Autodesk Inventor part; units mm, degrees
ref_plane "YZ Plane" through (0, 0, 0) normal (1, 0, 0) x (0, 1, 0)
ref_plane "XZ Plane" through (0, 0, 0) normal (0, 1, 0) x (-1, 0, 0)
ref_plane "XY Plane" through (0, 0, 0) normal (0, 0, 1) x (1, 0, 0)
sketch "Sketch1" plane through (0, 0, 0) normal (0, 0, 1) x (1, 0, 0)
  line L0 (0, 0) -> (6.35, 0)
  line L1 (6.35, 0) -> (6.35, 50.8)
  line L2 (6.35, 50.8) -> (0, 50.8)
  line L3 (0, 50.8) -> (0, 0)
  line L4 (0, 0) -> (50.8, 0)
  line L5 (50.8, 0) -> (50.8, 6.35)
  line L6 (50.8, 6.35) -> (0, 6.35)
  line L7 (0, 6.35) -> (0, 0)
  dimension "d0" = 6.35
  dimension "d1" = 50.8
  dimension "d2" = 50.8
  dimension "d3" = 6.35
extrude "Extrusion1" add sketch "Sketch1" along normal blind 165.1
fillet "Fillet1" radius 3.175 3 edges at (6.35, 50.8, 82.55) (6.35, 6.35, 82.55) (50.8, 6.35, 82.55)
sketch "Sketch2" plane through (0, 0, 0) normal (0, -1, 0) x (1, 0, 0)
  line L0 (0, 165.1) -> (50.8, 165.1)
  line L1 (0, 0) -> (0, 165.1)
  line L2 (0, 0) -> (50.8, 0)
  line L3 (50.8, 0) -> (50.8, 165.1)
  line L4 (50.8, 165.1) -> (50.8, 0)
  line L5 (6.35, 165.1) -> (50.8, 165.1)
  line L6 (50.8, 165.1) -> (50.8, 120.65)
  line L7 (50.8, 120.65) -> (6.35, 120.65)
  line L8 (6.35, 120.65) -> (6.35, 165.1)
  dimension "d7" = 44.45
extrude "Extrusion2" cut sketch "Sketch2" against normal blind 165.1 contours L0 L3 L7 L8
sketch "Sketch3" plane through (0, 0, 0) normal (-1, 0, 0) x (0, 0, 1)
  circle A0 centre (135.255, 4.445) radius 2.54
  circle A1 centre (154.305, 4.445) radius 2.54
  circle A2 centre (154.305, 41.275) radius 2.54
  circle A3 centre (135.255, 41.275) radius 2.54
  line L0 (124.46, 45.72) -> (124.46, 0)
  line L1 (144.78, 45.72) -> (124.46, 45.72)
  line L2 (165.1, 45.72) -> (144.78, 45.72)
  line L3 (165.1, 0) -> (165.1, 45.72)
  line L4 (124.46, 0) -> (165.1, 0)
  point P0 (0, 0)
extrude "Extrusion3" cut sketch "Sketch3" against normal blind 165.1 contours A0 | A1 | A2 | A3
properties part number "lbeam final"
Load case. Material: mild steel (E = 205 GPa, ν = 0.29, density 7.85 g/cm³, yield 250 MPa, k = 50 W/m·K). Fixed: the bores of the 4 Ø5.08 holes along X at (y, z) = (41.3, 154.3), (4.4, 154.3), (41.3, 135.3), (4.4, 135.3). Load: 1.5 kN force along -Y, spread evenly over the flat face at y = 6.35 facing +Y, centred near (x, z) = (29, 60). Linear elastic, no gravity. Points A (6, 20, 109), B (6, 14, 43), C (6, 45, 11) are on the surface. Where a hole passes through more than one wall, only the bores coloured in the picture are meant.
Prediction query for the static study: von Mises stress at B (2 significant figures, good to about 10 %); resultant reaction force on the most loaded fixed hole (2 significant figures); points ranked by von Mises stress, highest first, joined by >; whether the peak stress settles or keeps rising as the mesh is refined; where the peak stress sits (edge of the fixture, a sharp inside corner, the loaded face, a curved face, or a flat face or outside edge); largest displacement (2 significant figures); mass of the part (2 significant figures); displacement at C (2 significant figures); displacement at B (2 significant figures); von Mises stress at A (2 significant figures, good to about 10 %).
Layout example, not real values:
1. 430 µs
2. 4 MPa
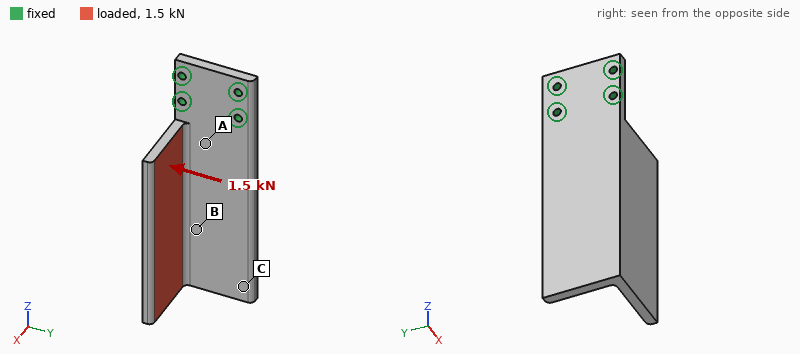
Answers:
1. 32 MPa
2. 2.9 kN
3. A > B > C
4. keeps rising
5. edge of the fixture
6. 0.38 mm
7. 680 g
8. 0.064 mm
9. 0.083 mm
10. 76 MPa
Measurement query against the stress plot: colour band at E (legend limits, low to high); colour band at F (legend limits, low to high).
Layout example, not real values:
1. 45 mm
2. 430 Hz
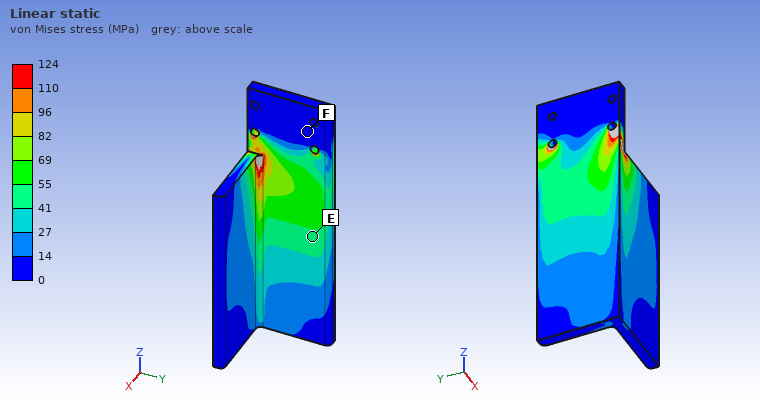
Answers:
1. 41 to 55 MPa
2. 0 to 14 MPa
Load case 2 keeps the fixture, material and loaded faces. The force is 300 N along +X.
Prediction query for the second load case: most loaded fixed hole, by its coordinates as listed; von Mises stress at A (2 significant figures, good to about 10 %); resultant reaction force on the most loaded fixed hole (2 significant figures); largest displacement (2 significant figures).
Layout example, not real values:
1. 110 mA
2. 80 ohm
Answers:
1. (4.4, 135.3)
2. 30 MPa
3. 450 N
4. 0.34 mm
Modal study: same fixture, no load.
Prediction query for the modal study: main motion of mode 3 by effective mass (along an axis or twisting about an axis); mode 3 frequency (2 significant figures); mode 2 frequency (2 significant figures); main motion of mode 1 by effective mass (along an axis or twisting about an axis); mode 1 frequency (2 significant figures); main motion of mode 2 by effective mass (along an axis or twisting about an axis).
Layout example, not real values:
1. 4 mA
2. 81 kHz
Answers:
1. along Y
2. 1700 Hz
3. 790 Hz
4. along X
5. 250 Hz
6. along Y
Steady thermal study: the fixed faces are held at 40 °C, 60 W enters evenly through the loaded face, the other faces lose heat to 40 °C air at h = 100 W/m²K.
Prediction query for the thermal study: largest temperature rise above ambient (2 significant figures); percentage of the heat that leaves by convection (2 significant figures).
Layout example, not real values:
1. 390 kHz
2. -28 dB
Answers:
1. 46 K
2. 88 %
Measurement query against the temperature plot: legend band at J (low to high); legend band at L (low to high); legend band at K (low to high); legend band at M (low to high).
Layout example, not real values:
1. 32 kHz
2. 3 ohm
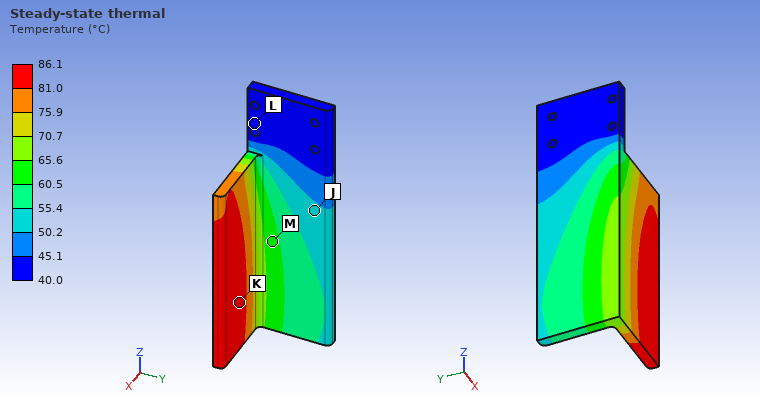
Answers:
1. 50.2 to 55.4 °C
2. 40.0 to 45.1 °C
3. 81.0 to 86.1 °C
4. 60.5 to 65.6 °C
